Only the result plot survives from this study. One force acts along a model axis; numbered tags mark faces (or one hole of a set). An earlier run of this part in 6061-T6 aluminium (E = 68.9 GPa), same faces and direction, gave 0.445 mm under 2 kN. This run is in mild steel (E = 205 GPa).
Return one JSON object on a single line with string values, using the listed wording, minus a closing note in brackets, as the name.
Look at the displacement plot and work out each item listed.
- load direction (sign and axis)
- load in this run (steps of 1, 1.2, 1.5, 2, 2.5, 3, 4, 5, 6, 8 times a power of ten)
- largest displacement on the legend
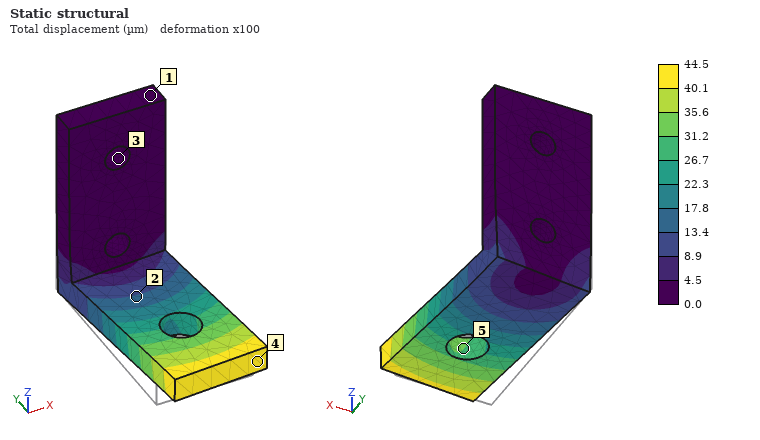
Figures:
{"load direction": "+X", "load in this run": "600 N", "largest displacement on the legend": "44.5 µm"}
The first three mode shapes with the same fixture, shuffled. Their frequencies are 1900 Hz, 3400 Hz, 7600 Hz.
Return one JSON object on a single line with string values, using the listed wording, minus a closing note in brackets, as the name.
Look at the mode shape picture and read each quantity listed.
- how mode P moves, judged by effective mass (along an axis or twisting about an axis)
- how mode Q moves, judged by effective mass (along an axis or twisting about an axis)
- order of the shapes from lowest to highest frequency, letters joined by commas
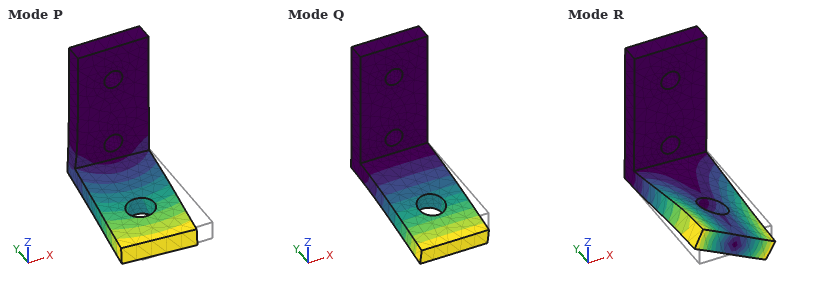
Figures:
{"how mode P moves, judged by effective mass": "along X", "how mode Q moves, judged by effective mass": "along Z", "order of the shapes from lowest to highest frequency, letters joined by commas": "Q, P, R"}
